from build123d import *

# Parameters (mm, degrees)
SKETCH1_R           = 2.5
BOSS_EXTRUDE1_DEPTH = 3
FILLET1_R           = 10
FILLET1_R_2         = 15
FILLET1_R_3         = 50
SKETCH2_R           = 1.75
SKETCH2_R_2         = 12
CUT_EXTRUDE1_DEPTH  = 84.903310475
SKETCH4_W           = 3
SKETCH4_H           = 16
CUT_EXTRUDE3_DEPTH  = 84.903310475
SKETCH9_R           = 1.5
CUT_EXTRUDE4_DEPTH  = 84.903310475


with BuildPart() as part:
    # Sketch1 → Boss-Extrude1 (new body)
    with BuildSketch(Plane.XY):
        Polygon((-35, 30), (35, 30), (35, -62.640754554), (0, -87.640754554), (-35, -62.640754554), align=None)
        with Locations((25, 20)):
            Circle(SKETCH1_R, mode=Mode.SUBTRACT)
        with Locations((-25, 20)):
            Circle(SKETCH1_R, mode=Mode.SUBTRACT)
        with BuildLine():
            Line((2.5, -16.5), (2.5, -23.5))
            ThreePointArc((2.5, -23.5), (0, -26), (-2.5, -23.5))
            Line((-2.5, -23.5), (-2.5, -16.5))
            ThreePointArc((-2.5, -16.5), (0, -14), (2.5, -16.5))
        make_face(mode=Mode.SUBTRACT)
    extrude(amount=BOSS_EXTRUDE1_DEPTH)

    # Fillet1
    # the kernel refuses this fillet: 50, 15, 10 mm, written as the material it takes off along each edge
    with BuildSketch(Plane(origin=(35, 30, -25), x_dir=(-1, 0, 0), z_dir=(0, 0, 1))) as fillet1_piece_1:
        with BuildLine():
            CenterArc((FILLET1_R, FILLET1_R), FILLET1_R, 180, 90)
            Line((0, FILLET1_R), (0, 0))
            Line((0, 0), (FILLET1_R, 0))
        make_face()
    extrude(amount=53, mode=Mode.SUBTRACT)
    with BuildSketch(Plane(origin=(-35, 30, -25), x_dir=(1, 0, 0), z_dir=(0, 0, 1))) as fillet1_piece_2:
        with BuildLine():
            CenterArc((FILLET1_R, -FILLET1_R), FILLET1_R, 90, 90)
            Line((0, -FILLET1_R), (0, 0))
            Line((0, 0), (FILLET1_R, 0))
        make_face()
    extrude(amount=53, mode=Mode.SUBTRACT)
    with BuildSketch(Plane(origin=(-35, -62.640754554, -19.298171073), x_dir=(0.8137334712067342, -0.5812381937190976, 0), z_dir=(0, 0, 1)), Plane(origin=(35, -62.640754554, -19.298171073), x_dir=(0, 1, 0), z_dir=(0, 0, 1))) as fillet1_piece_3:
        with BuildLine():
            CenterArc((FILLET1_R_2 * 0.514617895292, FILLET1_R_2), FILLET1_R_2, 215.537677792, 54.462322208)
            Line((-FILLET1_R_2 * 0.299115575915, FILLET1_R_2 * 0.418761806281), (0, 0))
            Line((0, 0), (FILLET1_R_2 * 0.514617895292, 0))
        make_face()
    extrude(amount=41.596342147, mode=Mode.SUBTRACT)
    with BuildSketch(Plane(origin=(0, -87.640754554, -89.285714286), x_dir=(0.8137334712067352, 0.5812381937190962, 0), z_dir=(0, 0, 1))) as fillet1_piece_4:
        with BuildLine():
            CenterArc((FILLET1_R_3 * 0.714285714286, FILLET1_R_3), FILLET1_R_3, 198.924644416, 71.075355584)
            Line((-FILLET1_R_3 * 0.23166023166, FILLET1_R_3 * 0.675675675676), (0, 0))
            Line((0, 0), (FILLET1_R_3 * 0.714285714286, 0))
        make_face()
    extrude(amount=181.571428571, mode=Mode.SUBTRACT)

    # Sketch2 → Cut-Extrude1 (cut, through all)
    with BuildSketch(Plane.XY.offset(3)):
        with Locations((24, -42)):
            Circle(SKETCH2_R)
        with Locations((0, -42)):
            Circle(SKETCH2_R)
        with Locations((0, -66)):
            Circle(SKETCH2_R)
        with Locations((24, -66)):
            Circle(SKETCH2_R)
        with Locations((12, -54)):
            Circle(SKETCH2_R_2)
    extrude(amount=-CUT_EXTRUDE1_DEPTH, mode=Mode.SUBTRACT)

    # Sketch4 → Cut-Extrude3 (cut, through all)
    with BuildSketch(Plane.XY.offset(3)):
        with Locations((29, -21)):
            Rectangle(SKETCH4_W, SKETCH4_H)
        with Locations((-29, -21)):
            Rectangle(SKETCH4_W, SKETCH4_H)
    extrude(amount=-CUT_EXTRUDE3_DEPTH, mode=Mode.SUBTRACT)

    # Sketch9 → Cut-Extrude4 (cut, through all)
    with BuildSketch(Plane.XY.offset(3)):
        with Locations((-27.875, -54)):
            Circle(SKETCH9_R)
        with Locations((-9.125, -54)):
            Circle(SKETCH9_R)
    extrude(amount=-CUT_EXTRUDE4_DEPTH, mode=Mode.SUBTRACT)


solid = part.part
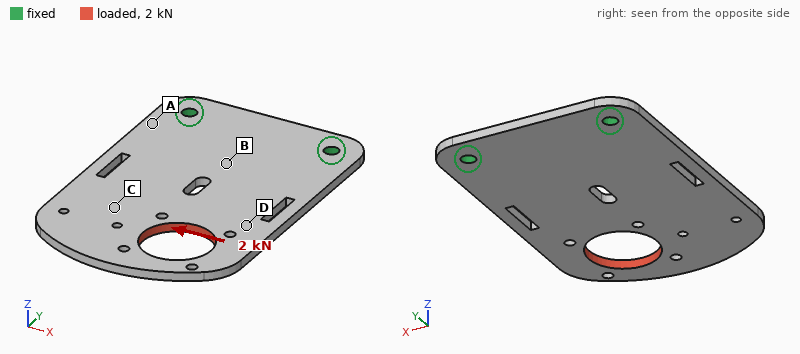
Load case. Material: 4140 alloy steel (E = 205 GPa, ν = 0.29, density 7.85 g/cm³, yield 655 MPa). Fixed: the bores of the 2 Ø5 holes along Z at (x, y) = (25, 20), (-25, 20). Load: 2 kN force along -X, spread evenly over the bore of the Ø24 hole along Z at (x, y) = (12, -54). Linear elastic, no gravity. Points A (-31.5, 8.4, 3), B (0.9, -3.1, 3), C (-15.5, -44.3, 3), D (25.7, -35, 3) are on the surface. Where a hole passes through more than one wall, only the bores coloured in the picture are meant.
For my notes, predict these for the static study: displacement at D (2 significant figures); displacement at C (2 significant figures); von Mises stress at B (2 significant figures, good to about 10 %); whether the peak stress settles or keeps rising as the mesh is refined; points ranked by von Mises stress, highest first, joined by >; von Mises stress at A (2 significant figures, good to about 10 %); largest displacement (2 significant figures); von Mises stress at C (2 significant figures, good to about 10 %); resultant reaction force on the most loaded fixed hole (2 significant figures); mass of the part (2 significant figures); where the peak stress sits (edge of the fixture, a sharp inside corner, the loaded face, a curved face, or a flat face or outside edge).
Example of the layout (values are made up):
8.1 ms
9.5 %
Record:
24 µm
27 µm
30 MPa
keeps rising
A > B > C > D
42 MPa
44 µm
15 MPa
3.0 kN
150 g
edge of the fixture
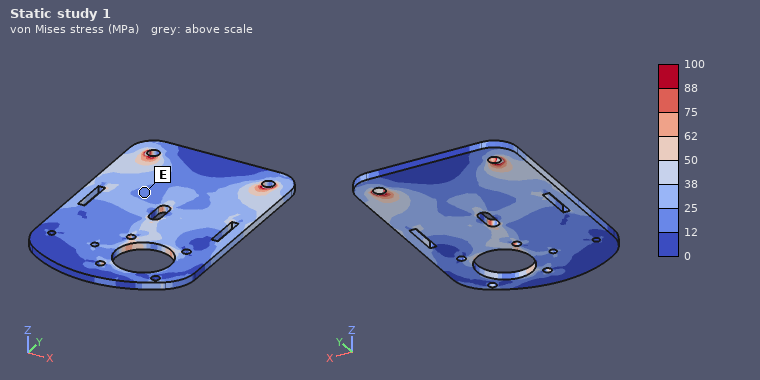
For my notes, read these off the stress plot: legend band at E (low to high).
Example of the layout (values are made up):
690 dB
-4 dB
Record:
12 to 25 MPa
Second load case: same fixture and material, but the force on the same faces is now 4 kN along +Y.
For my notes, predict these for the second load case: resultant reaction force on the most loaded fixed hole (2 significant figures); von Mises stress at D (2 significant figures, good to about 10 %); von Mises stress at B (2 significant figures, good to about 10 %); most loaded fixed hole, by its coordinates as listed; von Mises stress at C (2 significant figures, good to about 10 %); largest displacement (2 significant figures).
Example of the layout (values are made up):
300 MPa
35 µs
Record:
3.0 kN
32 MPa
11 MPa
(25, 20)
12 MPa
25 µm
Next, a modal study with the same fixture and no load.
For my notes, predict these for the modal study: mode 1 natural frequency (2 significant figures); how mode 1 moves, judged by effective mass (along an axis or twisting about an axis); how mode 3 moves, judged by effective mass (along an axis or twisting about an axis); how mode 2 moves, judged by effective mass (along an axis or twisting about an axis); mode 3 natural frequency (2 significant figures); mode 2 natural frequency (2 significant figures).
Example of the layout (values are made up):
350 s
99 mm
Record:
310 Hz
along Z
along Z
twisting about Y
1700 Hz
970 Hz
